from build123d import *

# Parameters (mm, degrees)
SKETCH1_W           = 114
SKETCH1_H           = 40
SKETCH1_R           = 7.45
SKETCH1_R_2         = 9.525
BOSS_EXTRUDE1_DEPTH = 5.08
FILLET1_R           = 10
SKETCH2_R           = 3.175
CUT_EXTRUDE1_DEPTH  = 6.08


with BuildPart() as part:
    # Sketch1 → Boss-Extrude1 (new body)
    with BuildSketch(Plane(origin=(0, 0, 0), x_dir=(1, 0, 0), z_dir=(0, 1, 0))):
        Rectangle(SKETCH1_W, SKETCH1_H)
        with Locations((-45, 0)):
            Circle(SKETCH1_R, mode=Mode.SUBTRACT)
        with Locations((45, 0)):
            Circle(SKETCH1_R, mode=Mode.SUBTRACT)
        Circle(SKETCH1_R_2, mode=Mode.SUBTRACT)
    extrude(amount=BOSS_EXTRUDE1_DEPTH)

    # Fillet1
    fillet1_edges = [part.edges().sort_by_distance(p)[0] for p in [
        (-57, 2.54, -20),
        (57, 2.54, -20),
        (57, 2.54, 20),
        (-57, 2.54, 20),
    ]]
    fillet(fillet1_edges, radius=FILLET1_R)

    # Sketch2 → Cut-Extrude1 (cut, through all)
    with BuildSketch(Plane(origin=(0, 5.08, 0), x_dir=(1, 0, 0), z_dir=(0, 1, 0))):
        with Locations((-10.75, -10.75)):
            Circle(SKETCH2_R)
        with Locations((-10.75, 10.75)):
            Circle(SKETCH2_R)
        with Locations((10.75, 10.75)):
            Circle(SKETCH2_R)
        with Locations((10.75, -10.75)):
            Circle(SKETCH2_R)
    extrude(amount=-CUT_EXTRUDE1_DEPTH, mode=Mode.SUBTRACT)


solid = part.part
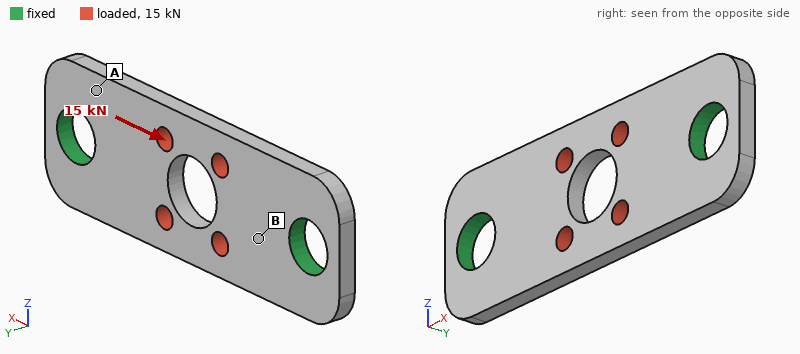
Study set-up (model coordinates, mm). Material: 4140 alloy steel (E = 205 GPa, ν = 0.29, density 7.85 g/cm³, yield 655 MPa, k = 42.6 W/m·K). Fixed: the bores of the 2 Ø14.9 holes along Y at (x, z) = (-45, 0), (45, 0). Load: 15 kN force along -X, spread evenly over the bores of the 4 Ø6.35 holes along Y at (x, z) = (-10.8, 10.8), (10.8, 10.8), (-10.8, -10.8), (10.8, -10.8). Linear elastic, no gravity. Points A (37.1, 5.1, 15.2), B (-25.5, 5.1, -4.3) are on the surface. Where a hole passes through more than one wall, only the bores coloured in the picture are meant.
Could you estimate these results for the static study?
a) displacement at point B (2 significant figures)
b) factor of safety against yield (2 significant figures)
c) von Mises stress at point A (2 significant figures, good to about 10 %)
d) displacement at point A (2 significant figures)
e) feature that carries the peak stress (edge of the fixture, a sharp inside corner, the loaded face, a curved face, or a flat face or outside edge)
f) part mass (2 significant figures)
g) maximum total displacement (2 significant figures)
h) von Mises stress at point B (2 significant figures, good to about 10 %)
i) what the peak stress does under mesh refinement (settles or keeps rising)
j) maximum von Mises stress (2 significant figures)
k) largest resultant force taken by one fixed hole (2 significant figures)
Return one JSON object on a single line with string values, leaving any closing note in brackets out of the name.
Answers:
{"displacement at point B": "3.3 µm", "factor of safety against yield": "4.4", "von Mises stress at point A": "23 MPa", "displacement at point A": "2.7 µm", "feature that carries the peak stress": "the loaded face", "part mass": "150 g", "maximum total displacement": "9.9 µm", "von Mises stress at point B": "45 MPa", "what the peak stress does under mesh refinement": "settles", "maximum von Mises stress": "150 MPa", "largest resultant force taken by one fixed hole": "7.5 kN"}
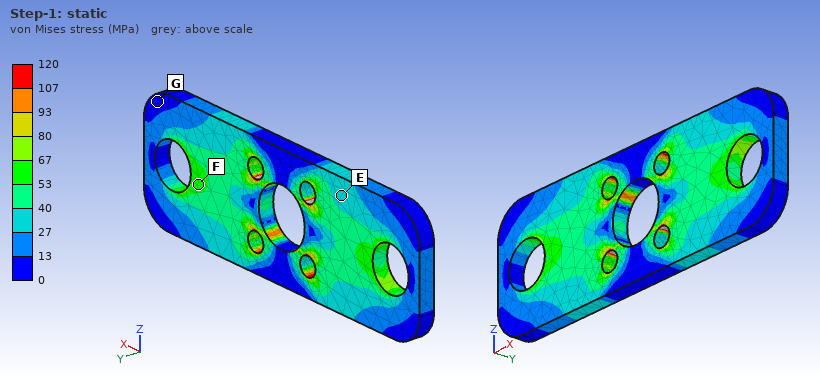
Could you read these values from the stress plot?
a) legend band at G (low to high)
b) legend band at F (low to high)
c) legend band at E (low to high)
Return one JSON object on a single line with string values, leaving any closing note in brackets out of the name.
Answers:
{"legend band at G": "0 to 13 MPa", "legend band at F": "53 to 67 MPa", "legend band at E": "27 to 40 MPa"}
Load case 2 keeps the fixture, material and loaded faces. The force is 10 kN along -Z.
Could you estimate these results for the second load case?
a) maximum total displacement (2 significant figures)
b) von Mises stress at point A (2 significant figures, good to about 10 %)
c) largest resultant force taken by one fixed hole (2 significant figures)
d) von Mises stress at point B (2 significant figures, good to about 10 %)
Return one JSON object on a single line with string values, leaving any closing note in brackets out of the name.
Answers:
{"maximum total displacement": "22 µm", "von Mises stress at point A": "26 MPa", "largest resultant force taken by one fixed hole": "5.0 kN", "von Mises stress at point B": "57 MPa"}
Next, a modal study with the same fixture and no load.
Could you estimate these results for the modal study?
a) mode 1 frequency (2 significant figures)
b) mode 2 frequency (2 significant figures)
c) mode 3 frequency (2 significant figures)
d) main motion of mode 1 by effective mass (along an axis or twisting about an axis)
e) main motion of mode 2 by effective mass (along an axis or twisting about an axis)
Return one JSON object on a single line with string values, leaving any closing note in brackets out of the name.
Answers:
{"mode 1 frequency": "4100 Hz", "mode 2 frequency": "5500 Hz", "mode 3 frequency": "9400 Hz", "main motion of mode 1 by effective mass": "along Y", "main motion of mode 2 by effective mass": "twisting about X"}
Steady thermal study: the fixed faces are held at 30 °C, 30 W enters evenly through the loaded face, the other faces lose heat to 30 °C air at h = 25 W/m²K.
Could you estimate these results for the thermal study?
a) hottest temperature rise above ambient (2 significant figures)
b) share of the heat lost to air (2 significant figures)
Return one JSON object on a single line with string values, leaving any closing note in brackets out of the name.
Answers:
{"hottest temperature rise above ambient": "55 K", "share of the heat lost to air": "17 %"}
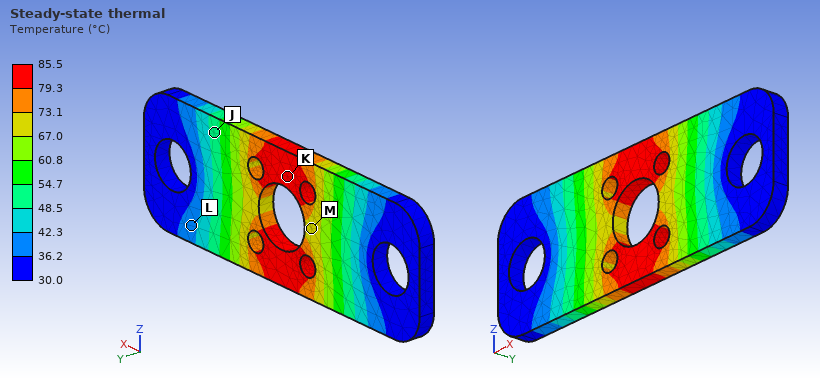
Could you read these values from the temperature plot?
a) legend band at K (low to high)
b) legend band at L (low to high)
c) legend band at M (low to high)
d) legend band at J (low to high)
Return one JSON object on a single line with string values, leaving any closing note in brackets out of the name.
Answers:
{"legend band at K": "79.3 to 85.5 °C", "legend band at L": "36.2 to 42.3 °C", "legend band at M": "67.0 to 73.1 °C", "legend band at J": "48.5 to 54.7 °C"}
